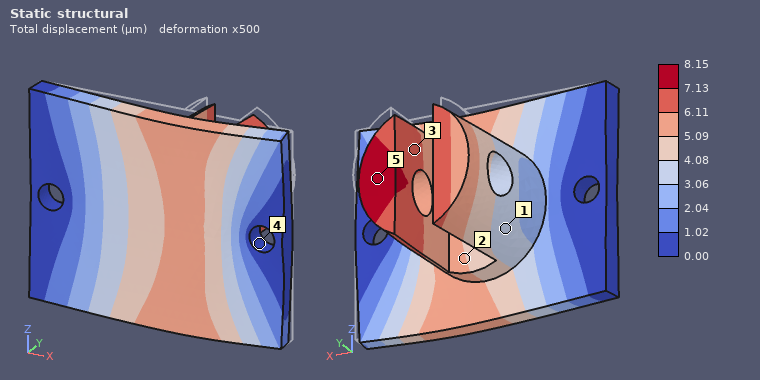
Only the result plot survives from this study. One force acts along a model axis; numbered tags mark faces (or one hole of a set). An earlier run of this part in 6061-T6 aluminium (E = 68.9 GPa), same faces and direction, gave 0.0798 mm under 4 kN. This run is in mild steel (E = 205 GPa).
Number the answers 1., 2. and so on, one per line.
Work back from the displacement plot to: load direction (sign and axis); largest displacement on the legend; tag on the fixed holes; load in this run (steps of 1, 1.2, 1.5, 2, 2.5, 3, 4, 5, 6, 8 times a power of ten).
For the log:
1. -Y
2. 8.15 µm
3. 4
4. 1.2 kN
